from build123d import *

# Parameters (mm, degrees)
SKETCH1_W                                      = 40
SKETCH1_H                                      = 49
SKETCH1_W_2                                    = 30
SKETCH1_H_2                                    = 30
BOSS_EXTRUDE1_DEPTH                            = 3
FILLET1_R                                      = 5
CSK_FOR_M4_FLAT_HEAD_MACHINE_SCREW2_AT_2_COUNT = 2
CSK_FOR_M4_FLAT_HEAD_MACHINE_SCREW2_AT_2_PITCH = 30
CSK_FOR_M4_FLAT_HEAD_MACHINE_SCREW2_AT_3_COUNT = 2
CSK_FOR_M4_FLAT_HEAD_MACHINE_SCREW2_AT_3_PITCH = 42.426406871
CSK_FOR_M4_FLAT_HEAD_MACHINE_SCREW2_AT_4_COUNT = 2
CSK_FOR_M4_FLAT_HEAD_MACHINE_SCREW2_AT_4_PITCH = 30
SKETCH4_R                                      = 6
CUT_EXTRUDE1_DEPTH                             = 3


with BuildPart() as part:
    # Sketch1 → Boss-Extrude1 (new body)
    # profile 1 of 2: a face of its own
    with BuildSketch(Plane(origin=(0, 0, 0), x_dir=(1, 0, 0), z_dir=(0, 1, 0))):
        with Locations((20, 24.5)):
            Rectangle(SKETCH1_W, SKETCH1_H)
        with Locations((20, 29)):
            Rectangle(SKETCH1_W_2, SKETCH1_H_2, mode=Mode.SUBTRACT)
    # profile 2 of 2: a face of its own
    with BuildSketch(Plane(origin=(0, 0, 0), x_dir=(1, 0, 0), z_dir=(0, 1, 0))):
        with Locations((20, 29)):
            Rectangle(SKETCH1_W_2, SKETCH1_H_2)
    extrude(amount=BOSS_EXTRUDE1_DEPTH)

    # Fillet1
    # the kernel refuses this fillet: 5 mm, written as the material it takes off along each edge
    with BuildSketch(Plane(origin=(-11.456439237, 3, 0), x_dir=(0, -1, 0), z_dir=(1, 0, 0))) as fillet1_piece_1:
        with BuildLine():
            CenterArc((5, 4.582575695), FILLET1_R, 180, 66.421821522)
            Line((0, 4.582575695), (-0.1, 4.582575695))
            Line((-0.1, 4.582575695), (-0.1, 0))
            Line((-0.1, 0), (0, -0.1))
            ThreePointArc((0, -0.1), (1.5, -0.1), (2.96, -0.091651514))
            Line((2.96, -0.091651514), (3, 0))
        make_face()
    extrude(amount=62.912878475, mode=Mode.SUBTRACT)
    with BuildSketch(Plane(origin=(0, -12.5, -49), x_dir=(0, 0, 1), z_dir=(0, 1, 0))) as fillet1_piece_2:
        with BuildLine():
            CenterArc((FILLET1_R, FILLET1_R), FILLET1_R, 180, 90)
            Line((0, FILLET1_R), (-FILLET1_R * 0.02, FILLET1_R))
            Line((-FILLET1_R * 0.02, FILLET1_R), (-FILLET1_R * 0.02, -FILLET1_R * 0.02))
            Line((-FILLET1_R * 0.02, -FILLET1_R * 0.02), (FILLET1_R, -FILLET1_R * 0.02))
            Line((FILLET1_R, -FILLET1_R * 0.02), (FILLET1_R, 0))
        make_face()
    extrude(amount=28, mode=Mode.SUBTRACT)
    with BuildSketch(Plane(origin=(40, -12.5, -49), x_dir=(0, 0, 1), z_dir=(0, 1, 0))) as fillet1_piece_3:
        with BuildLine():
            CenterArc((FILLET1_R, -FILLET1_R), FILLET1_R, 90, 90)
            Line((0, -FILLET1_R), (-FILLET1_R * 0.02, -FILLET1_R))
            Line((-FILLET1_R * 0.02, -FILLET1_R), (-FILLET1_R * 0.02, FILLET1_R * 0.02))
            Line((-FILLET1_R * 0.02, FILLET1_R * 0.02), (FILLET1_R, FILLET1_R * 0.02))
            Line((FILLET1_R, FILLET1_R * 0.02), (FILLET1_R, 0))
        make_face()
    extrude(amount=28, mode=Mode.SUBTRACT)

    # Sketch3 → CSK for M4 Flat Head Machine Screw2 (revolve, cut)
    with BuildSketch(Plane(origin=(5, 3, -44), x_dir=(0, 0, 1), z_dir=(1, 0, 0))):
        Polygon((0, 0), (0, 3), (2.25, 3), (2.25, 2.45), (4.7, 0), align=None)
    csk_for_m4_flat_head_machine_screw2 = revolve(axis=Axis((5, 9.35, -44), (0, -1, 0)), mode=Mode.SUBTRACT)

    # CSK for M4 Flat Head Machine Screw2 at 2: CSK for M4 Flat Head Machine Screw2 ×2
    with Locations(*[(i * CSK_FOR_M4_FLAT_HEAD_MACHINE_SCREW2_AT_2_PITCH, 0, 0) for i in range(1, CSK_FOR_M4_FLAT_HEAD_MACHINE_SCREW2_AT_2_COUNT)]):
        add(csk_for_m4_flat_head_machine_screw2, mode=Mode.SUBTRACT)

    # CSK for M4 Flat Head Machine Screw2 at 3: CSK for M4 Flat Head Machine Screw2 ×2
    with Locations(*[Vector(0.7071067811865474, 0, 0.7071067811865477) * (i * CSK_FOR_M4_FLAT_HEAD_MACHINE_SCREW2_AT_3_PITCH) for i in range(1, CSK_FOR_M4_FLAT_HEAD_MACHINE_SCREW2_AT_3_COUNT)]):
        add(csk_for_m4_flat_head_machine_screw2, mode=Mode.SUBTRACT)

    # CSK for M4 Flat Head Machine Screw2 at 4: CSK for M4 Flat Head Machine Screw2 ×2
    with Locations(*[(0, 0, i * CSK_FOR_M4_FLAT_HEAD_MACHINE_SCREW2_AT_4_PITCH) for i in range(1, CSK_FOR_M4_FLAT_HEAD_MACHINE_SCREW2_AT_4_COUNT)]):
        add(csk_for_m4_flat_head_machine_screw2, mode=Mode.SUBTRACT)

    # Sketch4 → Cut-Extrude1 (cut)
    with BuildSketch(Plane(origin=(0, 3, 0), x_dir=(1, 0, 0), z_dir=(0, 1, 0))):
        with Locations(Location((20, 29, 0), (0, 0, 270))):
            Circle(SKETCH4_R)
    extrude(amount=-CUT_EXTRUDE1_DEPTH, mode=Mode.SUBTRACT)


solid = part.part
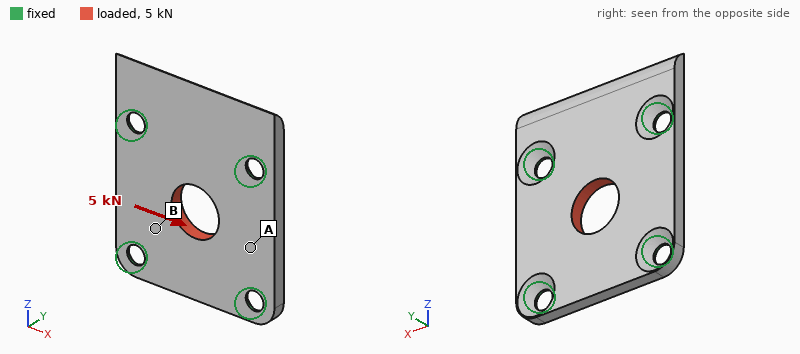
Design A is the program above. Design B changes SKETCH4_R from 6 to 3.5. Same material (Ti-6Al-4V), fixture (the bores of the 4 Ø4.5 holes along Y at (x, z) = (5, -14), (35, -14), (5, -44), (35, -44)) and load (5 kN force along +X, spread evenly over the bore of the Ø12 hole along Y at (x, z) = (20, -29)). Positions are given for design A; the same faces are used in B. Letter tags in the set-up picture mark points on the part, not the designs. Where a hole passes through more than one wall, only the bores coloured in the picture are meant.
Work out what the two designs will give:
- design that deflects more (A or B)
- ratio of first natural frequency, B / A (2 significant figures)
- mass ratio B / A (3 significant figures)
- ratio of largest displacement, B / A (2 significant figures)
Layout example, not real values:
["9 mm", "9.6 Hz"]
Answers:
["B", "1.0", "1.05", "1.1"]
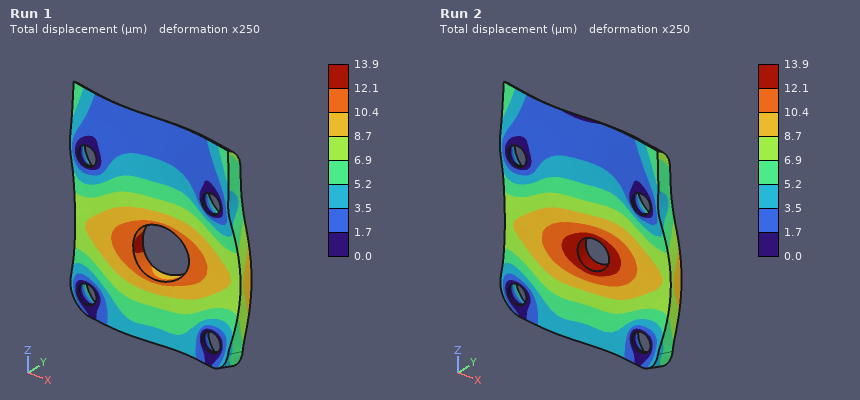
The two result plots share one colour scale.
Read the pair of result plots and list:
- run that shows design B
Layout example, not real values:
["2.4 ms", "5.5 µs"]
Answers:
["Run 2"]
